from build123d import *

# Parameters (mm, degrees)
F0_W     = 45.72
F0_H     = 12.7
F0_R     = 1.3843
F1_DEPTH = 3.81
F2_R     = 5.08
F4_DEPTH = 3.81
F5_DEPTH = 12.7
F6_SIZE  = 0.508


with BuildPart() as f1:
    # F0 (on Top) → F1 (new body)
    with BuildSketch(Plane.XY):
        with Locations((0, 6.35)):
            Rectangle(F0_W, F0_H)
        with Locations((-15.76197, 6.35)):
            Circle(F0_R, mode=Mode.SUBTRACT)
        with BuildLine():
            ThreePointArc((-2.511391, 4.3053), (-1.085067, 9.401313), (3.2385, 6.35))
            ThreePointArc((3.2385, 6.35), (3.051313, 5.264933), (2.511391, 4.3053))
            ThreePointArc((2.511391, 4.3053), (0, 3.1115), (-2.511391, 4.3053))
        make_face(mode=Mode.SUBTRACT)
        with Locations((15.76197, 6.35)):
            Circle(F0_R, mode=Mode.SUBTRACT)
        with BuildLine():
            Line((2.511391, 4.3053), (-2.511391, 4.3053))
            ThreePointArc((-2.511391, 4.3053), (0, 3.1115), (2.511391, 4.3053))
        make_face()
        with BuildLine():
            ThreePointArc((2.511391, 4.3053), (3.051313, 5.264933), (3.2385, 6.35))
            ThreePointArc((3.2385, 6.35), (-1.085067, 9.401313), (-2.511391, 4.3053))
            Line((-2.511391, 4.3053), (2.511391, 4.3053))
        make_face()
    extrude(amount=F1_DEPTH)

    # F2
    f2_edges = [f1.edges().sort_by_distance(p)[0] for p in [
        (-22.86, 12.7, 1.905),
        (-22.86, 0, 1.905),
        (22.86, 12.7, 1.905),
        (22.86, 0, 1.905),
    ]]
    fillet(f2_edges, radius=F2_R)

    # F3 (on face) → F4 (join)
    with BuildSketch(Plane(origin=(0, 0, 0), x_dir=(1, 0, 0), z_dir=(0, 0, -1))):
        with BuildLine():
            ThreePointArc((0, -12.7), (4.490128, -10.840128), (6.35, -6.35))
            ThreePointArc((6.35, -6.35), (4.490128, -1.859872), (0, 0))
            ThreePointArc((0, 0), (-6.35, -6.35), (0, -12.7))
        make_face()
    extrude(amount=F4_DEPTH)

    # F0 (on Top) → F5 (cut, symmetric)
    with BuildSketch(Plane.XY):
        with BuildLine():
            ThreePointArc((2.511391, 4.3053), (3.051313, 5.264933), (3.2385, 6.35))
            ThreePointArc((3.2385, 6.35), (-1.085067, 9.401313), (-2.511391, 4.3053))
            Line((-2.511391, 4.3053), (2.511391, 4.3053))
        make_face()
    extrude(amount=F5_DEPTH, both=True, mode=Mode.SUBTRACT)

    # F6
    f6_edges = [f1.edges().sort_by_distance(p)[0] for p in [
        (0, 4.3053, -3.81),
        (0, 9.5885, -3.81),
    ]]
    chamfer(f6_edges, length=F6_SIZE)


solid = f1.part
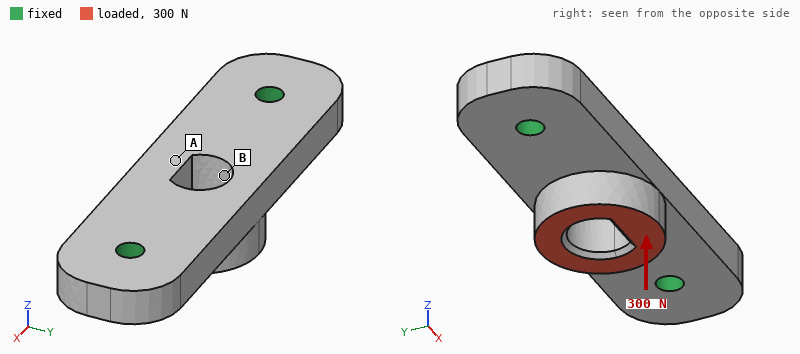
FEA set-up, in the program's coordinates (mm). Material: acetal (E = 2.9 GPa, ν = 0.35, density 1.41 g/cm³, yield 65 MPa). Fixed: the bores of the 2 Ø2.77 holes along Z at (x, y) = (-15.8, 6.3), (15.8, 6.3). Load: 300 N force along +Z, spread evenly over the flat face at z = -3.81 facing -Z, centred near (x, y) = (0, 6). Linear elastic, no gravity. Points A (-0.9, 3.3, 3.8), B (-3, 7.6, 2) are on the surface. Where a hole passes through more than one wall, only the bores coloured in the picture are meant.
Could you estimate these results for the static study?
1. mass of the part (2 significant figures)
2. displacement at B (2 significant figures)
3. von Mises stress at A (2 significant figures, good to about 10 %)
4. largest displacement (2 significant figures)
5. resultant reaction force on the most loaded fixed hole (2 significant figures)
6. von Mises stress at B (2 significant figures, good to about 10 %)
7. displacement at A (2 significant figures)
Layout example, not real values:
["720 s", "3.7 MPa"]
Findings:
["3.3 g", "0.20 mm", "15 MPa", "0.23 mm", "170 N", "6.2 MPa", "0.21 mm"]
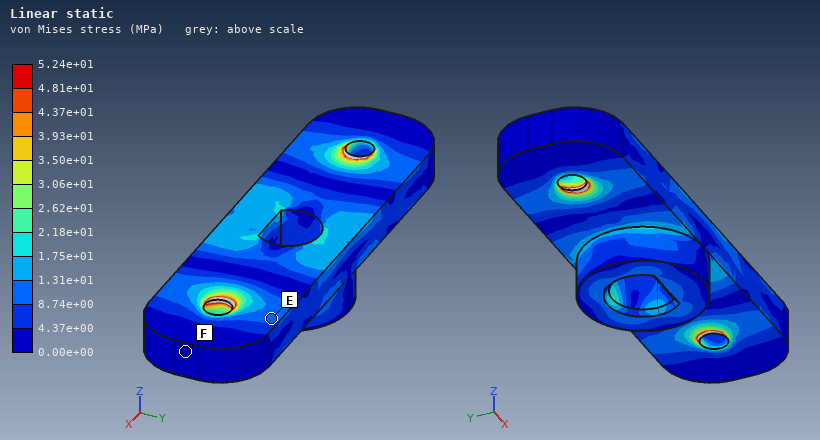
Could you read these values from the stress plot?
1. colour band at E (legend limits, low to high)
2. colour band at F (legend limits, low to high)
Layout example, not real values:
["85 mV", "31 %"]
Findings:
["8.74e+00 to 1.31e+01 MPa", "0.00e+00 to 4.37e+00 MPa"]
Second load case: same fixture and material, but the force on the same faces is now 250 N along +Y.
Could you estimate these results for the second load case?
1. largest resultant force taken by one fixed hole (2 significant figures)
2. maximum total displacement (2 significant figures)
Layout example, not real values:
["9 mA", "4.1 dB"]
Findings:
["130 N", "0.38 mm"]
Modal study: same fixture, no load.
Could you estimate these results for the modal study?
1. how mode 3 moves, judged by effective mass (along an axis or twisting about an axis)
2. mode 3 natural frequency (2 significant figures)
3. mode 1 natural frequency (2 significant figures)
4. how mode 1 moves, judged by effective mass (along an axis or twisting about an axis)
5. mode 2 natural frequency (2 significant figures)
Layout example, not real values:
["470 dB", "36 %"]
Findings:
["along Y", "8000 Hz", "5000 Hz", "along Z", "5400 Hz"]
